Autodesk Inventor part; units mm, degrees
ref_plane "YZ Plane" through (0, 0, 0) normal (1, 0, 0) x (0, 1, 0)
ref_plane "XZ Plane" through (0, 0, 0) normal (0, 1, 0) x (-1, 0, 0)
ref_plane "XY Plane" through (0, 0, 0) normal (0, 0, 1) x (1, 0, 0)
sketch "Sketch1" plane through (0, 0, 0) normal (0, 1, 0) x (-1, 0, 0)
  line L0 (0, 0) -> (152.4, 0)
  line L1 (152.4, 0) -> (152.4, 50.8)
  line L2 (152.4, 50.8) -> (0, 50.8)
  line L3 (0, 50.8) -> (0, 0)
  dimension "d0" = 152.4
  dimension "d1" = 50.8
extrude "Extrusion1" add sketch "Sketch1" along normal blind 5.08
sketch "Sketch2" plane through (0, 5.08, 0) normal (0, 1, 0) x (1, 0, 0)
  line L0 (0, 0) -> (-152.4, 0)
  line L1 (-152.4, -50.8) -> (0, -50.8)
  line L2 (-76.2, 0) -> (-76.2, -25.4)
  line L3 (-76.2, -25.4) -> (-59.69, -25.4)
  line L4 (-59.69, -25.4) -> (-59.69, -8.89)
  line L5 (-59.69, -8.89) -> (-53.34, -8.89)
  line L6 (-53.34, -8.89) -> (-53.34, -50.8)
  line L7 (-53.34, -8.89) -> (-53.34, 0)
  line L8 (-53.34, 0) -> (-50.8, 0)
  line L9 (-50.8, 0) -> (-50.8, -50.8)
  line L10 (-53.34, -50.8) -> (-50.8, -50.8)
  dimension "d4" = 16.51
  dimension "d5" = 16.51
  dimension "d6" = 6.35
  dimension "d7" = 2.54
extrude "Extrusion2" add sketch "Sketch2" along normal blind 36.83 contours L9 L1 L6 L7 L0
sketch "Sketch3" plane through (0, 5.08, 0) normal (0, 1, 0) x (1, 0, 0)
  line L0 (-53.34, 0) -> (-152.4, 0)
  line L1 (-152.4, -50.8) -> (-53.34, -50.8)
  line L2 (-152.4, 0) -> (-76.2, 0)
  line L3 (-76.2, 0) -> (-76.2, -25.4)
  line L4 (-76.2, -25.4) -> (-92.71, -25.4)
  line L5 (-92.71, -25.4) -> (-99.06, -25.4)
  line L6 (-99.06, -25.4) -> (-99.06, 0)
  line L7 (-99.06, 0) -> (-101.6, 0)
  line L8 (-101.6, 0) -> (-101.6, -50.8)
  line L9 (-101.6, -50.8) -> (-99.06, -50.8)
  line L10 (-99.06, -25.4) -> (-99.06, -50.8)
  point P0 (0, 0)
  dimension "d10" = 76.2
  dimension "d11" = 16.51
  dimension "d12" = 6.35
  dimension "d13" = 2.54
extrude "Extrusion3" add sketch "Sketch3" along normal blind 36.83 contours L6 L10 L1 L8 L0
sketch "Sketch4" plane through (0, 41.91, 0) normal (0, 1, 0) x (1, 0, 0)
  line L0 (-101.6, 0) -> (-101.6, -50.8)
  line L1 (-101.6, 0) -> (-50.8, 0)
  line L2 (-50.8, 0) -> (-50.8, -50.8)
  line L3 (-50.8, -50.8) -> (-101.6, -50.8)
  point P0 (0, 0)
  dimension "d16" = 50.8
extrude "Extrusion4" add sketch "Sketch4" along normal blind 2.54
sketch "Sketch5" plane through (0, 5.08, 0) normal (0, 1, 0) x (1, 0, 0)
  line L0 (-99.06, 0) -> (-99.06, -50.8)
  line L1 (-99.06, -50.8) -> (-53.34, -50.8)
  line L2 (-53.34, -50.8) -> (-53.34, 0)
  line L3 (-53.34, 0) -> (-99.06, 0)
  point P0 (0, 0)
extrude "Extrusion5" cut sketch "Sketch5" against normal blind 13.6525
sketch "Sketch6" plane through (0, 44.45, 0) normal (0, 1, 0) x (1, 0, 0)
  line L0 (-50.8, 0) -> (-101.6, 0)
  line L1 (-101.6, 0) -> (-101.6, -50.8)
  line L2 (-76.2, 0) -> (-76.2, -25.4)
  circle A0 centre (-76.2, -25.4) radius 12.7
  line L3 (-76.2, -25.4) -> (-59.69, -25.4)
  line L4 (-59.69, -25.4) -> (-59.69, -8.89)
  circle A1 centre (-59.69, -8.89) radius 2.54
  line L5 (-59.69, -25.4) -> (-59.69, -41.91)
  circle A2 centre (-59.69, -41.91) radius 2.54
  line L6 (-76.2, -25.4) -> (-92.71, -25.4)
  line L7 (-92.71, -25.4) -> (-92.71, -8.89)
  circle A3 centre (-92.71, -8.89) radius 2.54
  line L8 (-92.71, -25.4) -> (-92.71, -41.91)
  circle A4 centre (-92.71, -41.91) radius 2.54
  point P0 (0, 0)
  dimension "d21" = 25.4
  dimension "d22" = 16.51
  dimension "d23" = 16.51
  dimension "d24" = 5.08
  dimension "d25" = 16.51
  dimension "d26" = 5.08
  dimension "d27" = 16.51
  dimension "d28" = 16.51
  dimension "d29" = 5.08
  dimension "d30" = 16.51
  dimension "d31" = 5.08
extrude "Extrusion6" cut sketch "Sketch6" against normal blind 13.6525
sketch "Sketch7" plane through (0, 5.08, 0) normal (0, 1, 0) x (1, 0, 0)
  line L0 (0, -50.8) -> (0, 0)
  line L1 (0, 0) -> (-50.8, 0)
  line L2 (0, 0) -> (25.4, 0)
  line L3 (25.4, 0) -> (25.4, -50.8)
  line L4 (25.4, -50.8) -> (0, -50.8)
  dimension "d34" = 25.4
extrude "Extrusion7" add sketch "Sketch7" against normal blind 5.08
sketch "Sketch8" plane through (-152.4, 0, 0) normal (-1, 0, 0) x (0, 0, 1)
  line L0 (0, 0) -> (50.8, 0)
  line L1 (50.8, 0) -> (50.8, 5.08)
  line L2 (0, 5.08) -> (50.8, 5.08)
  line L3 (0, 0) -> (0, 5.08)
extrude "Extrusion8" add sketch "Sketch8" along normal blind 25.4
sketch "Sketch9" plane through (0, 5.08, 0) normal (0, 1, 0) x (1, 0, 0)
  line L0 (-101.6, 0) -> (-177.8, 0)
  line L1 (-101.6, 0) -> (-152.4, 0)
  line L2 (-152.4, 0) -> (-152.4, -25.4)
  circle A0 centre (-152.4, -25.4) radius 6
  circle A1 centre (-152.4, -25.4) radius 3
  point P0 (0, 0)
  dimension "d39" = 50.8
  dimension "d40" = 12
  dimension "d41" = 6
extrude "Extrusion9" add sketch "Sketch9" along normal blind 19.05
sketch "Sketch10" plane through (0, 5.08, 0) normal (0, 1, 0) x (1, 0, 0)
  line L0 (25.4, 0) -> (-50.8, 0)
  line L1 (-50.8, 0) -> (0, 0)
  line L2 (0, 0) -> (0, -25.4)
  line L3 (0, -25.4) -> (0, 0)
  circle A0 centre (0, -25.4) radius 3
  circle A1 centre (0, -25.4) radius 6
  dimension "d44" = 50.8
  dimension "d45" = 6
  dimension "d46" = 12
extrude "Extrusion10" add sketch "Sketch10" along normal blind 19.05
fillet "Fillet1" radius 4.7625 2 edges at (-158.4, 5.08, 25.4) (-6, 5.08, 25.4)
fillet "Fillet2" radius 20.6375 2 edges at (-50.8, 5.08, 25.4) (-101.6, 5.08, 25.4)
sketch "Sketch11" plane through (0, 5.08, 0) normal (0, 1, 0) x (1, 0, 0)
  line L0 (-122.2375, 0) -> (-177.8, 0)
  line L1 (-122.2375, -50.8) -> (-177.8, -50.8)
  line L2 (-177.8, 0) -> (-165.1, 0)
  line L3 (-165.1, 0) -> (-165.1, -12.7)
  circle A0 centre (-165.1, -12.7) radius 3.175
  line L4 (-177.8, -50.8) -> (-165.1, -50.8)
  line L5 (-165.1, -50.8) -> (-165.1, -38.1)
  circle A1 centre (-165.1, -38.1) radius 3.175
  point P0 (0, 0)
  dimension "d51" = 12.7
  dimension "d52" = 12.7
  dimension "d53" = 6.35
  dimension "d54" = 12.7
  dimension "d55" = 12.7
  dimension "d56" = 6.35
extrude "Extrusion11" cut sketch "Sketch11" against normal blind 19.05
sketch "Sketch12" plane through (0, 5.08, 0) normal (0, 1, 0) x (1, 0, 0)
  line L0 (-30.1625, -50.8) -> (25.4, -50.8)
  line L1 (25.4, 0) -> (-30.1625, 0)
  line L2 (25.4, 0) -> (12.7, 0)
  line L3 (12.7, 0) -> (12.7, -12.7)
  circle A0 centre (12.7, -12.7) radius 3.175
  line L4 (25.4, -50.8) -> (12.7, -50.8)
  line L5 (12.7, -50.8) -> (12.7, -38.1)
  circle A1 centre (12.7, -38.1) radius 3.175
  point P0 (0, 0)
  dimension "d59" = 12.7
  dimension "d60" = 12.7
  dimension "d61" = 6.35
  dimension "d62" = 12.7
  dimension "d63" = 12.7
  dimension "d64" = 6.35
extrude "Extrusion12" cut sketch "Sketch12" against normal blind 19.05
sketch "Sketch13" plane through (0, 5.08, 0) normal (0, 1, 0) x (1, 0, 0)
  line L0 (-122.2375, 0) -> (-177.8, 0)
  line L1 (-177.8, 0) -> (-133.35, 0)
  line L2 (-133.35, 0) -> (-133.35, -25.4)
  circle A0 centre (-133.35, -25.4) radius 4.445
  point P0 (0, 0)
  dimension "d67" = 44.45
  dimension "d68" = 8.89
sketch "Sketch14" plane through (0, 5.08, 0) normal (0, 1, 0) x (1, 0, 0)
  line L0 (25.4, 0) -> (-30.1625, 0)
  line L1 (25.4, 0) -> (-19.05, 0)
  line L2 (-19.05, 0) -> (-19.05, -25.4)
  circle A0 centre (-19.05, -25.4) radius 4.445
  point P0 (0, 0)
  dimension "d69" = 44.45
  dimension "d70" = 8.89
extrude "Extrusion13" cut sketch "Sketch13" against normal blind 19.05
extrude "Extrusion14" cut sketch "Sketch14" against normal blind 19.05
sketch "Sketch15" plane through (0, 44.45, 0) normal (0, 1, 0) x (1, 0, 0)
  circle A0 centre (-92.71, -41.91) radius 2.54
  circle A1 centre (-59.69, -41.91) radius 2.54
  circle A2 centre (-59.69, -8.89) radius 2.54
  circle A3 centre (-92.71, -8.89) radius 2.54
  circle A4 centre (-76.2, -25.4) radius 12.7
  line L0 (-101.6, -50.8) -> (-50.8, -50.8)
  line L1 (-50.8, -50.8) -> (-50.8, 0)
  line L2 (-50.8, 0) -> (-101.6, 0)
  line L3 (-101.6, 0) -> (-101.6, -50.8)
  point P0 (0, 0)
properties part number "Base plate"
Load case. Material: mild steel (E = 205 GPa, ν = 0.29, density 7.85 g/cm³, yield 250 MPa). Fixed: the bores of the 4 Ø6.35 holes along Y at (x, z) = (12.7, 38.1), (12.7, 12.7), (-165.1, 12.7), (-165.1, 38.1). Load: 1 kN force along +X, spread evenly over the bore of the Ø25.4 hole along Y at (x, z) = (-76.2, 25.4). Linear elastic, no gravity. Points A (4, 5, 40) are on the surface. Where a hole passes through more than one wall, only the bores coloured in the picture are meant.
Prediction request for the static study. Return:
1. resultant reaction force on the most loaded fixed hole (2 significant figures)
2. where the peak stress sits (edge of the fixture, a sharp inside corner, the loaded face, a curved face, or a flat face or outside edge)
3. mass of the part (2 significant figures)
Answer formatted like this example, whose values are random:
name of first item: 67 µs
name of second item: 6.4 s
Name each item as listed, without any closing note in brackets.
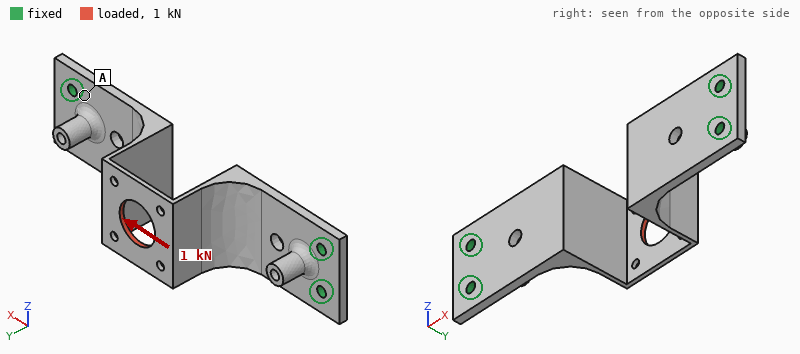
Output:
resultant reaction force on the most loaded fixed hole: 280 N
where the peak stress sits: a curved face
mass of the part: 530 g
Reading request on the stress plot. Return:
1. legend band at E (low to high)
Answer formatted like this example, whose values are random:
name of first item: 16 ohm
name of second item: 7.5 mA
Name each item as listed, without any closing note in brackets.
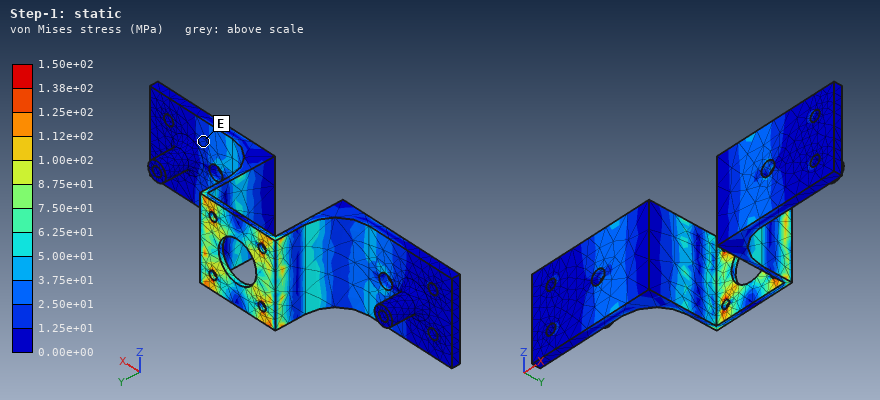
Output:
legend band at E: 1.25e+01 to 2.50e+01 MPa
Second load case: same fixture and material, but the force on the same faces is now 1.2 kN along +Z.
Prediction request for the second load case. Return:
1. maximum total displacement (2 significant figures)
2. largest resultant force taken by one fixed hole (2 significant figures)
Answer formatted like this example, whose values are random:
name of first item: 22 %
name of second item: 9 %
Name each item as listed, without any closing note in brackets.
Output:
maximum total displacement: 0.23 mm
largest resultant force taken by one fixed hole: 1.7 kN
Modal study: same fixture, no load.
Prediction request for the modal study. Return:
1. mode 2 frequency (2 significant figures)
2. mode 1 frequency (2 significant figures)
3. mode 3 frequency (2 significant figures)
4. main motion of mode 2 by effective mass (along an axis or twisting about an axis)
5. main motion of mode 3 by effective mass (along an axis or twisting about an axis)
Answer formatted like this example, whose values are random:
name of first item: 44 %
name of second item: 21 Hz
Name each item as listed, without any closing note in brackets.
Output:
mode 2 frequency: 900 Hz
mode 1 frequency: 840 Hz
mode 3 frequency: 1200 Hz
main motion of mode 2 by effective mass: along Y
main motion of mode 3 by effective mass: along Z
